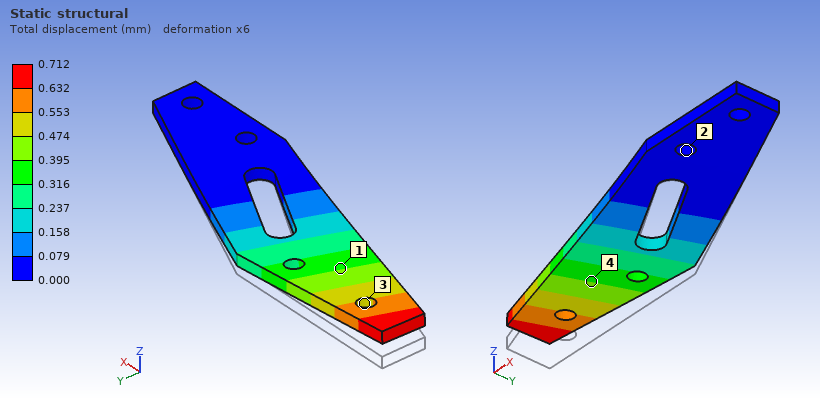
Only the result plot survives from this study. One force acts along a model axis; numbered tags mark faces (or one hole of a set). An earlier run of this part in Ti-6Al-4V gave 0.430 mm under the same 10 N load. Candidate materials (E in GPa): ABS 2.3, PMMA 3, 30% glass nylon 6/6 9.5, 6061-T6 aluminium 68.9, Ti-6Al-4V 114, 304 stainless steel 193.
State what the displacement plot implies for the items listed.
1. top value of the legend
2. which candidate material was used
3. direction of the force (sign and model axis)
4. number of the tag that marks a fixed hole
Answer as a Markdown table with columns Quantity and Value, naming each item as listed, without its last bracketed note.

| Quantity | Value |
|---|---|
| top value of the legend | 0.712 mm |
| which candidate material was used | 6061-T6 aluminium |
| direction of the force | +Z |
| number of the tag that marks a fixed hole | 2 |
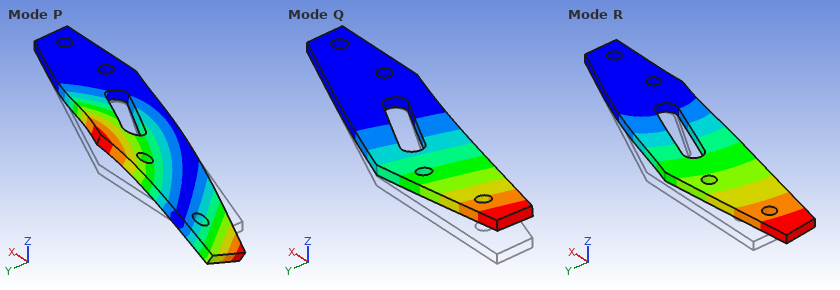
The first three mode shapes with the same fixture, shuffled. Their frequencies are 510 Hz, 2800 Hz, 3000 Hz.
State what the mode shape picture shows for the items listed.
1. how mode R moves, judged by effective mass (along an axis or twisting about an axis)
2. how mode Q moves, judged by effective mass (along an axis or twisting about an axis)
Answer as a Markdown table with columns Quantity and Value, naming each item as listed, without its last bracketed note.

| Quantity | Value |
|---|---|
| how mode R moves, judged by effective mass | along Y |
| how mode Q moves, judged by effective mass | along Z |
